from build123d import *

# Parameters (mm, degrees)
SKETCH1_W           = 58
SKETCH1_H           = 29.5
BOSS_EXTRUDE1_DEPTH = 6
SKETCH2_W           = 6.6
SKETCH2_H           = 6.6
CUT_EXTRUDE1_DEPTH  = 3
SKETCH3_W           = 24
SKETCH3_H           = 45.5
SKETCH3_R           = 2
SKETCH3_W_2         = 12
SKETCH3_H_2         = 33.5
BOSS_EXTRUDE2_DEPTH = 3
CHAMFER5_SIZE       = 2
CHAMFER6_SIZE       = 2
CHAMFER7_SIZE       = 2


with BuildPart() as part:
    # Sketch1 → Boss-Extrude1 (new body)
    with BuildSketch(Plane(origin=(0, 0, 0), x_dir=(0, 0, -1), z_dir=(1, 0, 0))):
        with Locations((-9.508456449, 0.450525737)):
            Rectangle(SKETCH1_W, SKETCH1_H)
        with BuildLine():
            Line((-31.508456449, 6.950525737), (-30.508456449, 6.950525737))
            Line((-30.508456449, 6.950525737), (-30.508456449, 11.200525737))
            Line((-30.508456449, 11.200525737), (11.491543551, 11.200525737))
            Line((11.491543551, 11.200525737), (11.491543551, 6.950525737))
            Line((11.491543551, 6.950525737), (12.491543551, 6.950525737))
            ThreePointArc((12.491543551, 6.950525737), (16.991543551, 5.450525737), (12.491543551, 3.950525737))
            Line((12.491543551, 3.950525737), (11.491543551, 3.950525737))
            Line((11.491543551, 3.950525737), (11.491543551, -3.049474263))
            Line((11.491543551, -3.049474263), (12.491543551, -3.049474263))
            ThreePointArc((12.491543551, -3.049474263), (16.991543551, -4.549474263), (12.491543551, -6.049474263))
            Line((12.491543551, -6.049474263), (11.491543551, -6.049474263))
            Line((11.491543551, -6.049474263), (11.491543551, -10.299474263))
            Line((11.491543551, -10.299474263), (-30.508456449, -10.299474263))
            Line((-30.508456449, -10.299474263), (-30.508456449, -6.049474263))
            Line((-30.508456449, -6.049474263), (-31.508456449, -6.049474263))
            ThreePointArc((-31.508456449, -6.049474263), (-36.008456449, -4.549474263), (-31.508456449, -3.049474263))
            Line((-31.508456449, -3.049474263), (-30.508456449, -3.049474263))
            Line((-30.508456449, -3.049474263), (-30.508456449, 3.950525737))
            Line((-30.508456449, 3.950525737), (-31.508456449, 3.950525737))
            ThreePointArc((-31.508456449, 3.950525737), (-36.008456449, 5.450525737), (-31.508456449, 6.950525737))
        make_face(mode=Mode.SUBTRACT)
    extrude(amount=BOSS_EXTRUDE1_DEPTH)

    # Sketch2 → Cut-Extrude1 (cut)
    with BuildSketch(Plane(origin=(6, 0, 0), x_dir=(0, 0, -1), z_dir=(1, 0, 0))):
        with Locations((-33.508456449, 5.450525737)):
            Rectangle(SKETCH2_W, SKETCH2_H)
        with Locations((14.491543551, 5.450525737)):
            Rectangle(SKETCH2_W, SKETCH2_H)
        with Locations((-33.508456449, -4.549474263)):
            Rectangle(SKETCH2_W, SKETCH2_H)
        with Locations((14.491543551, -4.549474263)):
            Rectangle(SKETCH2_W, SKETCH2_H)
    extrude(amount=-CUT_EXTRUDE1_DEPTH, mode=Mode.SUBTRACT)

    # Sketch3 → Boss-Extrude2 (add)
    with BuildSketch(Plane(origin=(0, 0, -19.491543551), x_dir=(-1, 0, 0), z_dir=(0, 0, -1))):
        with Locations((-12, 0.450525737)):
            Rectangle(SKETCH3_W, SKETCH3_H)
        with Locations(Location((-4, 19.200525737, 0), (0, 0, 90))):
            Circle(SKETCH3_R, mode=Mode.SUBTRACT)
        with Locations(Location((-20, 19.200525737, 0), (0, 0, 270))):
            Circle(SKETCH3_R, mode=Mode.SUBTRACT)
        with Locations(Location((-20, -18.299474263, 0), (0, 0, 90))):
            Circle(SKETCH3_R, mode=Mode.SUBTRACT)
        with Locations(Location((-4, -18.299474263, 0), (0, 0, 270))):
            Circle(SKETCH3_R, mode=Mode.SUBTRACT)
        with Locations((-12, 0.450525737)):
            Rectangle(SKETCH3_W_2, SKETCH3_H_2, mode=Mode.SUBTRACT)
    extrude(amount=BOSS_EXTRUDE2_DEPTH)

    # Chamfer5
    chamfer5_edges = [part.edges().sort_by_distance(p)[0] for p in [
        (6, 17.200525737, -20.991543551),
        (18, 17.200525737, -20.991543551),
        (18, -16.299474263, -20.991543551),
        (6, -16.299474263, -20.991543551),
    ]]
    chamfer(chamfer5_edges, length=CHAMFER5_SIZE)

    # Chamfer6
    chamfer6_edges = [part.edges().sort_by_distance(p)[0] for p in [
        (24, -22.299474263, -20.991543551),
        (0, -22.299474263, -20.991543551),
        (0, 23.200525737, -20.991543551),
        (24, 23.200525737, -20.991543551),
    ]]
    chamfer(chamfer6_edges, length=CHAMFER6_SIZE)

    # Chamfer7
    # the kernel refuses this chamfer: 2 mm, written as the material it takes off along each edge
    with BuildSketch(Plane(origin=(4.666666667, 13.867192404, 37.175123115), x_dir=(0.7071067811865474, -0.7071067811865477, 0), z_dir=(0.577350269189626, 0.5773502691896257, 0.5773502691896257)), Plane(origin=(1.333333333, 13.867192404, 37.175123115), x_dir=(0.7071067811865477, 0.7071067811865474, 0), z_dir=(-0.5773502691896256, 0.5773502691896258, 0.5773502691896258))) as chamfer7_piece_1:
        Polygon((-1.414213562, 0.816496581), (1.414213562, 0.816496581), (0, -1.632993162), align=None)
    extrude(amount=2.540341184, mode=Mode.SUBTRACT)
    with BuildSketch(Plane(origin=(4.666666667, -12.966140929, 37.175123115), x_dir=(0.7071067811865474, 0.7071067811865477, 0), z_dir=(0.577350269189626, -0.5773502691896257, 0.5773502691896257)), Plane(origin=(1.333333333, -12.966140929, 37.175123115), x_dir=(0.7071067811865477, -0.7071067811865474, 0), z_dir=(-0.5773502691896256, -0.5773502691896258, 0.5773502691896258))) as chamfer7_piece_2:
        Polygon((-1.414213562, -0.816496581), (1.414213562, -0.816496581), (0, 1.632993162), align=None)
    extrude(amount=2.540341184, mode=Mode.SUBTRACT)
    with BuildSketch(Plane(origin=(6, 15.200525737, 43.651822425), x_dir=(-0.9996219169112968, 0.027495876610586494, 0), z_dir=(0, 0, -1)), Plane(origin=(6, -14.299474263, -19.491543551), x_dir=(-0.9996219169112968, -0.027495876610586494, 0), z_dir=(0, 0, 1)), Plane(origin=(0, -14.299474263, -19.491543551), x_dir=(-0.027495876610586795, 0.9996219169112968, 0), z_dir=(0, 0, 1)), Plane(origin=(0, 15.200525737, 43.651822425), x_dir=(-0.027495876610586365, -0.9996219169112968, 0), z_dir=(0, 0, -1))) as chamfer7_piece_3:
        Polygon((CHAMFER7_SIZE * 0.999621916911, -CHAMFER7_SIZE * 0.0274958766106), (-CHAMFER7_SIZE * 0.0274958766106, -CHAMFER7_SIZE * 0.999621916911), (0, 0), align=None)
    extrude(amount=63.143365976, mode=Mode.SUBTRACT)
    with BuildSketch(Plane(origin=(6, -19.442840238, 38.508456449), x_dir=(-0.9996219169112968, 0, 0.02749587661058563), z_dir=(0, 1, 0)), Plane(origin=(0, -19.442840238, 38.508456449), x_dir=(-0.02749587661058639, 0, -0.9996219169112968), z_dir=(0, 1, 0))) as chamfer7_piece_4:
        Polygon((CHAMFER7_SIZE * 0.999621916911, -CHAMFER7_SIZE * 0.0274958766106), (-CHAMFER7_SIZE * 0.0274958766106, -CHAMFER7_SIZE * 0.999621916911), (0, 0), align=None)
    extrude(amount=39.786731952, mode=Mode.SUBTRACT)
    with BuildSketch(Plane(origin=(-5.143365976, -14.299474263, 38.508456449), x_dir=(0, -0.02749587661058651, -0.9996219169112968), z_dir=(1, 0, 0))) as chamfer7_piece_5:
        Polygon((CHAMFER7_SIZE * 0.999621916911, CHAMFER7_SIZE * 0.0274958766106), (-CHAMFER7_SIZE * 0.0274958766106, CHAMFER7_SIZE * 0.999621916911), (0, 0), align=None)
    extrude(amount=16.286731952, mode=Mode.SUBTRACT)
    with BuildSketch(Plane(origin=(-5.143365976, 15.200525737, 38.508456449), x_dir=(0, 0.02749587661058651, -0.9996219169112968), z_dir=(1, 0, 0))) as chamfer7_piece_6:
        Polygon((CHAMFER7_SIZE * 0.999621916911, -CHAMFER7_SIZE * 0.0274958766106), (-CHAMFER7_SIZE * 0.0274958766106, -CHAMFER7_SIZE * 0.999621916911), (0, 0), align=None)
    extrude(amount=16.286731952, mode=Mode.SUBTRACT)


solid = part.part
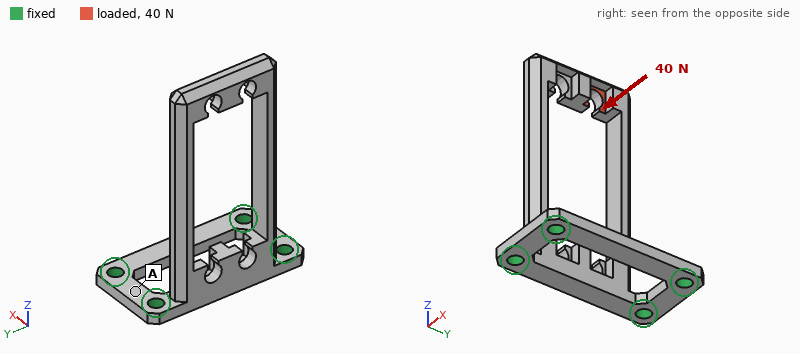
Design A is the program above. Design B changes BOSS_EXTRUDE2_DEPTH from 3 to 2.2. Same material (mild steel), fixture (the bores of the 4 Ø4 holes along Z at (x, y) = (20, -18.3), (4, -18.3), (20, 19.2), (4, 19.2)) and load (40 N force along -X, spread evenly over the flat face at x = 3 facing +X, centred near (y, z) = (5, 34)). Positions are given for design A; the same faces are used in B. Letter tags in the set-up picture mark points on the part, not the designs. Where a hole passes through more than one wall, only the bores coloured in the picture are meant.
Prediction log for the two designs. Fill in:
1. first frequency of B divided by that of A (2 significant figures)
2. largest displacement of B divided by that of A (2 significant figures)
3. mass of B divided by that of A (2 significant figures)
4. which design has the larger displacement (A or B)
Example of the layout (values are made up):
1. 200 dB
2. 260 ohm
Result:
1. 0.85
2. 1.3
3. 0.91
4. B
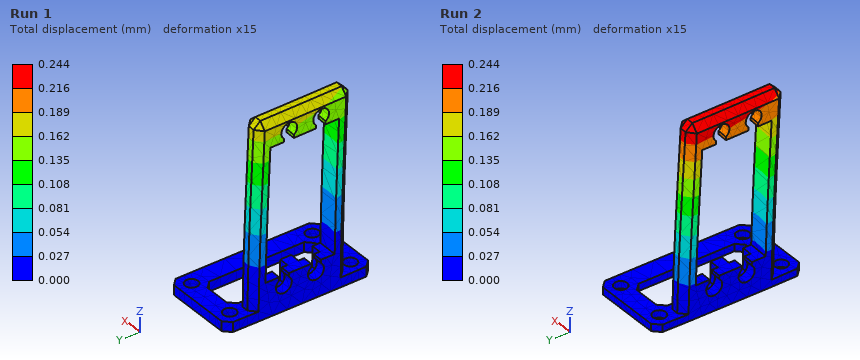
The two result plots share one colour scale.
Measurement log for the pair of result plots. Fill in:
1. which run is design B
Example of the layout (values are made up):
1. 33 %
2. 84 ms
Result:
1. Run 2
